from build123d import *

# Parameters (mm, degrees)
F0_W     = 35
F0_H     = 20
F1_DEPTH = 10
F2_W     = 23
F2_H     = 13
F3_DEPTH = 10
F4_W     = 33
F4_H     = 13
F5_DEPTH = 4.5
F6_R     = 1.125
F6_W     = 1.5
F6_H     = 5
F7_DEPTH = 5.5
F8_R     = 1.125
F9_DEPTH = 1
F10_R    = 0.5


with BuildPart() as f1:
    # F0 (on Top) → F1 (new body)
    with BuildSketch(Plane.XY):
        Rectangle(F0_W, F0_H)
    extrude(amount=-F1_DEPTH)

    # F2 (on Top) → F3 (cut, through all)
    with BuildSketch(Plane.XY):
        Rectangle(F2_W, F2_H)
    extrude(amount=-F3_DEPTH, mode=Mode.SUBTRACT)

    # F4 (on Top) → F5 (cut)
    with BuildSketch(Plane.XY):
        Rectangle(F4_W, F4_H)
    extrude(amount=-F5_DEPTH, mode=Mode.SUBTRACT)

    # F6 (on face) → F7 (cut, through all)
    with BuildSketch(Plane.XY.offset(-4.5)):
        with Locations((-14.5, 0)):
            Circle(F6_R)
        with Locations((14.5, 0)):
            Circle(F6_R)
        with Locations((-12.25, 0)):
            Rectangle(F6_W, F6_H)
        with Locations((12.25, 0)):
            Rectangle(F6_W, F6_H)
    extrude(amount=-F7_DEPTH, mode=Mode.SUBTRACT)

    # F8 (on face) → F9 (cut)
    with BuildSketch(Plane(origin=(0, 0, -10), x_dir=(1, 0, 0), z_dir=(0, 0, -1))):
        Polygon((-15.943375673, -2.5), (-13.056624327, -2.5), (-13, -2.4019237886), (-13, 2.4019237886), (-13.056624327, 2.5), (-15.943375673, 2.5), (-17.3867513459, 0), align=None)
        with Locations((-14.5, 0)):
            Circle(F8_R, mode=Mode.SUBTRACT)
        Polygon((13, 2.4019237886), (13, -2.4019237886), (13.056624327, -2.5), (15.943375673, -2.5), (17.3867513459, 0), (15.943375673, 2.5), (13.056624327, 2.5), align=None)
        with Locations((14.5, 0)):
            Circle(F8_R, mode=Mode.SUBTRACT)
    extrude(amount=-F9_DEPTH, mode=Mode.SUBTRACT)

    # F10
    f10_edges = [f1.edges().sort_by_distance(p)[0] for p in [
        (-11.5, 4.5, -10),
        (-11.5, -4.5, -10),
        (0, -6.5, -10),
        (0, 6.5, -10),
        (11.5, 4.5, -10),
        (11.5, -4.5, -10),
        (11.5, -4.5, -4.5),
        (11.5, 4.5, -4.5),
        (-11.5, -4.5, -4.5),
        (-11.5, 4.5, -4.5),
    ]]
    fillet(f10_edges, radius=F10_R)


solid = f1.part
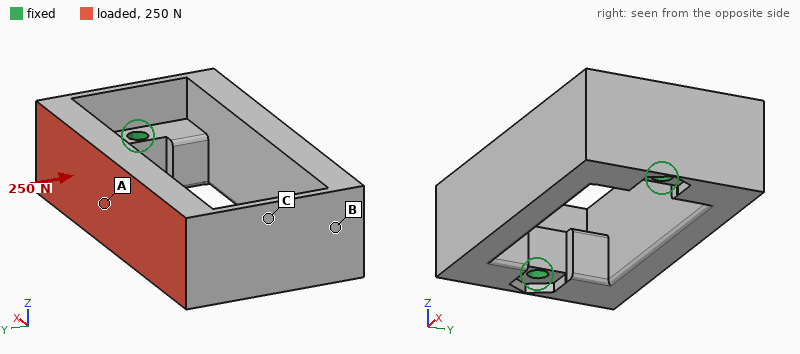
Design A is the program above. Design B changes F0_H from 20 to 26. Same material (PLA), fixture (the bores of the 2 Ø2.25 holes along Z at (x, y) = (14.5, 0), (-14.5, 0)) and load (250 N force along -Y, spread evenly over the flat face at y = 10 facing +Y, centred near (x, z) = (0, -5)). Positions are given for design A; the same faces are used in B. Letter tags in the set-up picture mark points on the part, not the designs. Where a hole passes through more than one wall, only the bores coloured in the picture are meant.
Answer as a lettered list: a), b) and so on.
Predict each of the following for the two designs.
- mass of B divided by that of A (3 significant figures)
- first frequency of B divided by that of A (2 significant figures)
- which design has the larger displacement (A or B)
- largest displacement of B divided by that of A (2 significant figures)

a) 1.64
b) 0.67
c) A
d) 0.51
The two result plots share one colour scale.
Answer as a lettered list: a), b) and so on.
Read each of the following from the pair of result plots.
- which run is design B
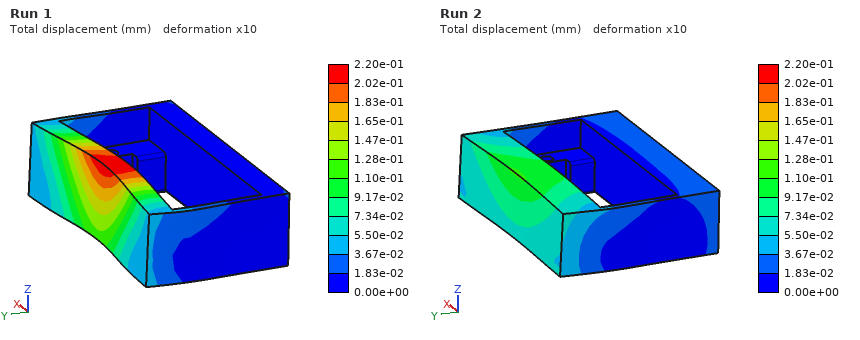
a) Run 2
